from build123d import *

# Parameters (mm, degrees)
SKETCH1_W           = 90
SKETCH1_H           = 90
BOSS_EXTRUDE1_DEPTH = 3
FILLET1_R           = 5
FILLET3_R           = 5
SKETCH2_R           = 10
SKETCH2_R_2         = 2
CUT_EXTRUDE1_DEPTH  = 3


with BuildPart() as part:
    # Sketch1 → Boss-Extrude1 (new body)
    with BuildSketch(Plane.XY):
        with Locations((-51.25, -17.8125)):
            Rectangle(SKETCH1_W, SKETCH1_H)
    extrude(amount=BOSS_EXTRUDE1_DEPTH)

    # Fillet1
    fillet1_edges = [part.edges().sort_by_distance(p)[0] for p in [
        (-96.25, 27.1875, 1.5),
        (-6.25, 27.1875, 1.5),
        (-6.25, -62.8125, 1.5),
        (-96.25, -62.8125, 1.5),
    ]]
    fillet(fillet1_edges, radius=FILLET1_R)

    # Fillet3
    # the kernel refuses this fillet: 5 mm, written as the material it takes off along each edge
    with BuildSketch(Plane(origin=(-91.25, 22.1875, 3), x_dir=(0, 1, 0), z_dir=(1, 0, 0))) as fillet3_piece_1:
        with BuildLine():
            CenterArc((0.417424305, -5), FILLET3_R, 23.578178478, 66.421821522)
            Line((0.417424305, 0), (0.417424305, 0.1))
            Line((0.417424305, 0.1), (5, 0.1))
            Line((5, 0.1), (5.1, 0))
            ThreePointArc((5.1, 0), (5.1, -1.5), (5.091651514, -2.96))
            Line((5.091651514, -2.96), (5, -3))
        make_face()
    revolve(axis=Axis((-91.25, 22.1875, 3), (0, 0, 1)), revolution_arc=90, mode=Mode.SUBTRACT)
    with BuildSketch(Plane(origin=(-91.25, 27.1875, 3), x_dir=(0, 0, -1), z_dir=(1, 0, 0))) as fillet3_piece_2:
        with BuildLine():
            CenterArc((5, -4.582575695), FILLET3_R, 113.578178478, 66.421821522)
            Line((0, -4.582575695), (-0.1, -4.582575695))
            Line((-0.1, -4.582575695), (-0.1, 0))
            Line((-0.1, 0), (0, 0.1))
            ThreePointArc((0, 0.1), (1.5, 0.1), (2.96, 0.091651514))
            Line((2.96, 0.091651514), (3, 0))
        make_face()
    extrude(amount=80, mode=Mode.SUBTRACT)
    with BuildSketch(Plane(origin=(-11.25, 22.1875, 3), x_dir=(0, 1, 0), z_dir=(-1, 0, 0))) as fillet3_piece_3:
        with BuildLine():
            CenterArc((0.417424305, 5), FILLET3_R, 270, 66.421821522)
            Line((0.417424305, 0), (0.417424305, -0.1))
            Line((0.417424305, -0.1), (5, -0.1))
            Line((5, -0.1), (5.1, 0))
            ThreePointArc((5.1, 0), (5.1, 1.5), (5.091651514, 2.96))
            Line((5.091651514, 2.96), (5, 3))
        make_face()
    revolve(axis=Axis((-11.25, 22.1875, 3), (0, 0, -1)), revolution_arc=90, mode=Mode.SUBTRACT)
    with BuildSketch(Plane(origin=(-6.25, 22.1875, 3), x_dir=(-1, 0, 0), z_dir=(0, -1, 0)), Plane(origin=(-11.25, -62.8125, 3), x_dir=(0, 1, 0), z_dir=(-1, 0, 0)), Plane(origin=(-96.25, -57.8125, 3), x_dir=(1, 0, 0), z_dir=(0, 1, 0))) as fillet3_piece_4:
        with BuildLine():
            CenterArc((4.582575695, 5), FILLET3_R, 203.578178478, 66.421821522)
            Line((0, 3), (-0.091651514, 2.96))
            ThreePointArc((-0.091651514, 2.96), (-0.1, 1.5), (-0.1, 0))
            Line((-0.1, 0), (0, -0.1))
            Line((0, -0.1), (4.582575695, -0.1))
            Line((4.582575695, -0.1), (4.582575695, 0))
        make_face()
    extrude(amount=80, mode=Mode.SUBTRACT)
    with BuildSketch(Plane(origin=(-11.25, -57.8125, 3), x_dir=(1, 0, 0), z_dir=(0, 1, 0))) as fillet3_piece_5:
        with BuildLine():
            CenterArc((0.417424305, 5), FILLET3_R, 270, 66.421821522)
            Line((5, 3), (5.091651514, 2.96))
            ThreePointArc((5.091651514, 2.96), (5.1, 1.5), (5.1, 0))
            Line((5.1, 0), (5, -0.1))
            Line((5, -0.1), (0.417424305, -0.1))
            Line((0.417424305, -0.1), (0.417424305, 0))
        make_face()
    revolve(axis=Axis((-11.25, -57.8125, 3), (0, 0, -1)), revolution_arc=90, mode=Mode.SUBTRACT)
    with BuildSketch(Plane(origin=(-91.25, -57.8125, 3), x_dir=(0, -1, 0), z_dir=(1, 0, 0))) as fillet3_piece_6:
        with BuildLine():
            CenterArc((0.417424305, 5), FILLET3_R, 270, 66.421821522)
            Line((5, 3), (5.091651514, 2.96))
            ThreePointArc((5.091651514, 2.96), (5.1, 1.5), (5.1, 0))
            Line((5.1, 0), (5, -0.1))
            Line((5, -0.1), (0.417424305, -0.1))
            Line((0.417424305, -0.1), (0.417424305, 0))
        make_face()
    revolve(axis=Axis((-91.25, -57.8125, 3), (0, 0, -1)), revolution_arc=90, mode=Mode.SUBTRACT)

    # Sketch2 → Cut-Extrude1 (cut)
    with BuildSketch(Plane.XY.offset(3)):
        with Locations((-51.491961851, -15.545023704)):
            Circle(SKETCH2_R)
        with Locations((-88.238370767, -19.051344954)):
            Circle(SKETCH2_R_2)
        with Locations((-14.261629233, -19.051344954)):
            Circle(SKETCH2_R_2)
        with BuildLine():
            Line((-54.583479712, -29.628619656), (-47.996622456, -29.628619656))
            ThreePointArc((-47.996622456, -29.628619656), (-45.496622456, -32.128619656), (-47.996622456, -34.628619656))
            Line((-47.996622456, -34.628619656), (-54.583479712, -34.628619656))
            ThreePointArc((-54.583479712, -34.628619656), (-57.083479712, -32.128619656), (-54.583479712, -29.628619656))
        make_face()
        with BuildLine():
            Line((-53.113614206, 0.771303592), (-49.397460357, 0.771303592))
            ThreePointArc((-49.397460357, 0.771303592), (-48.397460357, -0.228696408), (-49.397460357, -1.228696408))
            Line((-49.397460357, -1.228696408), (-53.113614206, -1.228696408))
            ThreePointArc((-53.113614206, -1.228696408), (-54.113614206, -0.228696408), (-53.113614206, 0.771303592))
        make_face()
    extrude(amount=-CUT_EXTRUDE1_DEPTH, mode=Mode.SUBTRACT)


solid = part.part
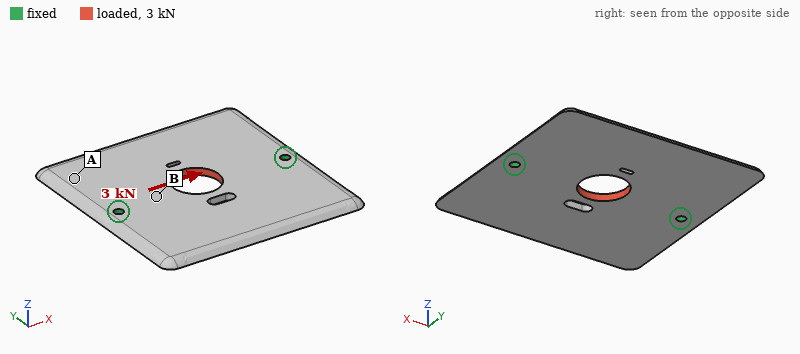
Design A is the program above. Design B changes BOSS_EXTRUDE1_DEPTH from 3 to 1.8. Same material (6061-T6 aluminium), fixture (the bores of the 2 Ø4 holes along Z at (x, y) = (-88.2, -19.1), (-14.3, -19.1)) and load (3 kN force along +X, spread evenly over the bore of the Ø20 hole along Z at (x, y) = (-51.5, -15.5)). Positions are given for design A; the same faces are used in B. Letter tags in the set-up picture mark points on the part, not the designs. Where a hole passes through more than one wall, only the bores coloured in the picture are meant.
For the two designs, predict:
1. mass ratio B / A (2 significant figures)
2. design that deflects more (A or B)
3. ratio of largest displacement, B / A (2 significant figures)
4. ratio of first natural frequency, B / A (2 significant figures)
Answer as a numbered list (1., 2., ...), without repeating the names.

1. 0.62
2. B
3. 1.6
4. 0.62
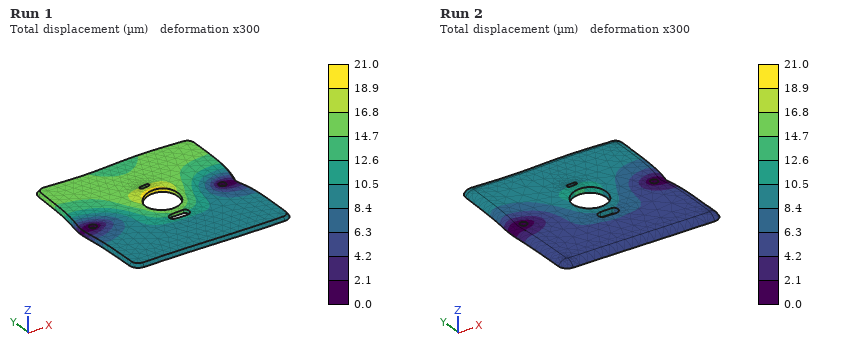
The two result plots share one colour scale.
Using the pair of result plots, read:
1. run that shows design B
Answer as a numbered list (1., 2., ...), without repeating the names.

1. Run 1
